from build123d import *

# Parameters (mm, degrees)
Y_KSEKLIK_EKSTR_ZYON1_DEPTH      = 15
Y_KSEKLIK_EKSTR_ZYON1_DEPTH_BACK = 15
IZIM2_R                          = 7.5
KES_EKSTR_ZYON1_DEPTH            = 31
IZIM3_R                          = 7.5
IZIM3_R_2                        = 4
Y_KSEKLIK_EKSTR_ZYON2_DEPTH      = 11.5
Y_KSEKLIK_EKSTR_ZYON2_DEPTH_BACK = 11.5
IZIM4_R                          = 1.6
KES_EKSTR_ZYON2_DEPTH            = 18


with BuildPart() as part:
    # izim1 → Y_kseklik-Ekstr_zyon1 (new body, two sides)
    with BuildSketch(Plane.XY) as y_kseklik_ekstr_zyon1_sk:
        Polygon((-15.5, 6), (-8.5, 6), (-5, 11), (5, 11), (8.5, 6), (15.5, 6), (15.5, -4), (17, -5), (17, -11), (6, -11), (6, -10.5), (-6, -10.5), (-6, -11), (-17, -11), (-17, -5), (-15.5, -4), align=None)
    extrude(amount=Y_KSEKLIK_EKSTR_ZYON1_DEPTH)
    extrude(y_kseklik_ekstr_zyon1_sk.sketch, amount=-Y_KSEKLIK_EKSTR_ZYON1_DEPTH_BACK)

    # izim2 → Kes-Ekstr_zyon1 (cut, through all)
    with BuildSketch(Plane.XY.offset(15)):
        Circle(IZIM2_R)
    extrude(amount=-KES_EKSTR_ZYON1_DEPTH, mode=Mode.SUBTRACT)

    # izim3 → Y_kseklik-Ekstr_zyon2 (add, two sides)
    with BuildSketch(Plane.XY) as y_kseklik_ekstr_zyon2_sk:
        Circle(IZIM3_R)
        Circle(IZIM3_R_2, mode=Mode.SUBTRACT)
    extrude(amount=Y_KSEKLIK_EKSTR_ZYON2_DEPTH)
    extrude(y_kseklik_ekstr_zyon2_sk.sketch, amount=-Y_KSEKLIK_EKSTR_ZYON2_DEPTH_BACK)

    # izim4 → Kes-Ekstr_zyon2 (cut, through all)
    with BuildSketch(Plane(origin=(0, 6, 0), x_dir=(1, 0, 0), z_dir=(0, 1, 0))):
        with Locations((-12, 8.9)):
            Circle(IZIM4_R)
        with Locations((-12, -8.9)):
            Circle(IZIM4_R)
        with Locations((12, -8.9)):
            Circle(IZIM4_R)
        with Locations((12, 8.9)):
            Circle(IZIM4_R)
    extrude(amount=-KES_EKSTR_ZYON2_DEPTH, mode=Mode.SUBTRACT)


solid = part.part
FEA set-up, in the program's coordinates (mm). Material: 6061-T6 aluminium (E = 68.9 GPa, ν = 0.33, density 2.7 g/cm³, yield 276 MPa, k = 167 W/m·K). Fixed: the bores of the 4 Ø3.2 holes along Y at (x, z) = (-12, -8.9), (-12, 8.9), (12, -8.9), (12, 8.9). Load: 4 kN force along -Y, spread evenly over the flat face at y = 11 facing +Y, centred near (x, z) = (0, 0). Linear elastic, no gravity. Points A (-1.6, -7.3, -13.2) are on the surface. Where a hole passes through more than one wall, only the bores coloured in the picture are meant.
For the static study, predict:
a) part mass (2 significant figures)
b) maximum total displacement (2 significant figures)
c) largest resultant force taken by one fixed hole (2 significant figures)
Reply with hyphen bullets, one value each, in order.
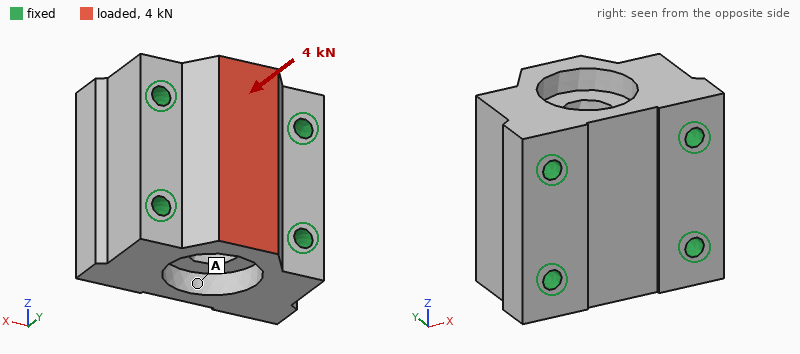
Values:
- 41 g
- 6.9 µm
- 1.1 kN
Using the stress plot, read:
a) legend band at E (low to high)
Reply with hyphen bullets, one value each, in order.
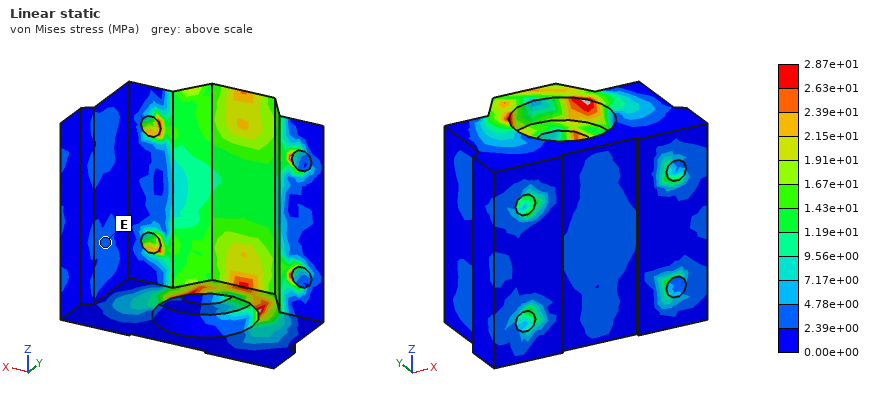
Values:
- 2.39e+00 to 4.78e+00 MPa
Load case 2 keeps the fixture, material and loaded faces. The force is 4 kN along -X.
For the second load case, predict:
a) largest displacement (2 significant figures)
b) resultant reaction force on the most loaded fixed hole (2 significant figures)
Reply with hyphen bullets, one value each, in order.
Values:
- 5.0 µm
- 1.3 kN
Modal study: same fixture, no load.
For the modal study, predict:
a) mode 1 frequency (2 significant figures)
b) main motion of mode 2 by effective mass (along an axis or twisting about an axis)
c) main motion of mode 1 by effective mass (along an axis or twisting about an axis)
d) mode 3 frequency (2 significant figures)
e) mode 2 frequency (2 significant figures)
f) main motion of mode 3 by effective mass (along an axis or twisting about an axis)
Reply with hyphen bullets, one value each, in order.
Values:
- 47 kHz
- along Y
- along Z
- 62 kHz
- 53 kHz
- along Z
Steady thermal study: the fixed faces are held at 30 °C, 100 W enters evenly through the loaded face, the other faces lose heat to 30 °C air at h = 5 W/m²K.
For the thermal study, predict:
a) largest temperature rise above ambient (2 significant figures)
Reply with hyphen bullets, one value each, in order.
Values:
- 24 K
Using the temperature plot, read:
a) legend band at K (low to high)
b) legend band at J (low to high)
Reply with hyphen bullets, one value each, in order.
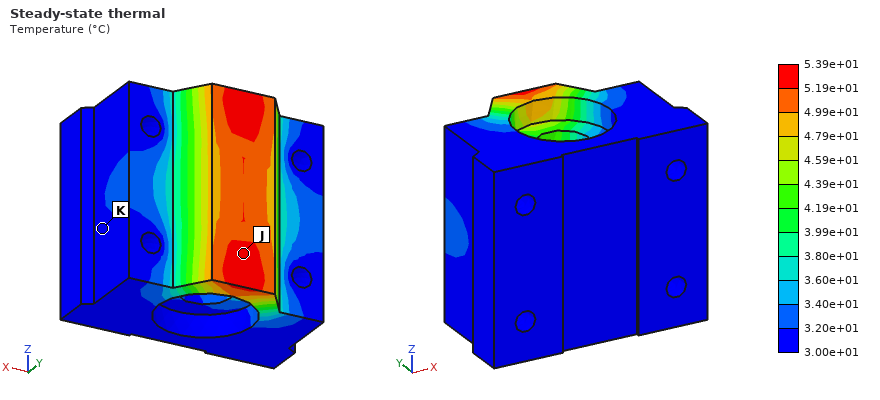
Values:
- 3.00e+01 to 3.20e+01 °C
- 5.19e+01 to 5.39e+01 °C
